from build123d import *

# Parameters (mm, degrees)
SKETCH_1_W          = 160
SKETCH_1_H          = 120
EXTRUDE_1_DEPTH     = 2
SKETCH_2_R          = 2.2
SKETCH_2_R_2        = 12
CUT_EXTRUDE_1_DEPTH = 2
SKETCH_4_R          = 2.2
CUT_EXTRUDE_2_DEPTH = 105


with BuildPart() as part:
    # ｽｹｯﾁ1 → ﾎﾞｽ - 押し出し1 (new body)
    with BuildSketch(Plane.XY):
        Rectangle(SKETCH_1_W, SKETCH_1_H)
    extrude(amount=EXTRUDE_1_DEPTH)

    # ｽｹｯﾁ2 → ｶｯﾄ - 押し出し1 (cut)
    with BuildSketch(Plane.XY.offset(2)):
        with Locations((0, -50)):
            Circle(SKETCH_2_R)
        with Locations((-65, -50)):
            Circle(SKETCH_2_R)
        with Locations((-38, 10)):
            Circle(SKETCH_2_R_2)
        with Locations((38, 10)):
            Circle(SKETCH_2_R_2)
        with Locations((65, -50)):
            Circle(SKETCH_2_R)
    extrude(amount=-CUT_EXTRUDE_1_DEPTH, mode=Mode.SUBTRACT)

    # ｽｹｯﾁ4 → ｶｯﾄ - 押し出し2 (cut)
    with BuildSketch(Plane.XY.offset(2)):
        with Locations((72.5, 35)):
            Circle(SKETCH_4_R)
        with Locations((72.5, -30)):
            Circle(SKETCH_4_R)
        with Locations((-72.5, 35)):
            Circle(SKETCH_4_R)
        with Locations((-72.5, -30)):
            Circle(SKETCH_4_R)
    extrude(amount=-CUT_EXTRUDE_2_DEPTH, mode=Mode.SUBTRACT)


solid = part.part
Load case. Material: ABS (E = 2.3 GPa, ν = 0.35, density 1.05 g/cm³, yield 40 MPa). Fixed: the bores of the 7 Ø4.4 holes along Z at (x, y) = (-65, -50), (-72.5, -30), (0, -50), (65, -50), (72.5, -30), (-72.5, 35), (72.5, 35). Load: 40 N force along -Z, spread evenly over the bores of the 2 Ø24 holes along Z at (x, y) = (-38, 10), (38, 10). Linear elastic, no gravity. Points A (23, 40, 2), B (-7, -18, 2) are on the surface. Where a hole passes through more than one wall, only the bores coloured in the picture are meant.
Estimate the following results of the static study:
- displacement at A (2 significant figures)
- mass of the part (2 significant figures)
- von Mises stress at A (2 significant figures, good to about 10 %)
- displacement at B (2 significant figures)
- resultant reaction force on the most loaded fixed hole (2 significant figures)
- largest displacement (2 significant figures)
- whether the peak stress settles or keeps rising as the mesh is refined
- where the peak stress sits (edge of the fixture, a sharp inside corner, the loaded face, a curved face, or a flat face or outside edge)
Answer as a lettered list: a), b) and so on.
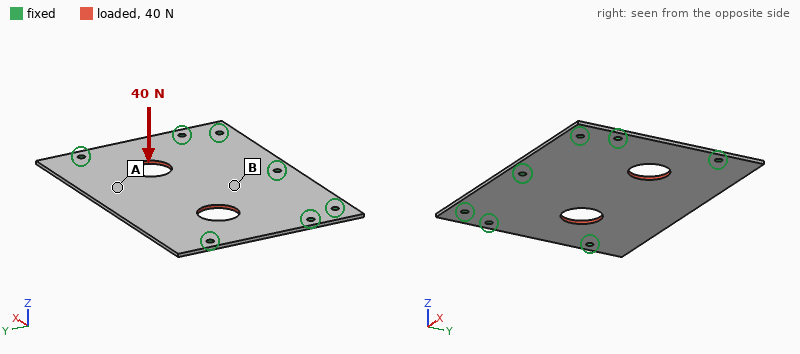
a) 1.7 mm
b) 38 g
c) 2.8 MPa
d) 1.0 mm
e) 12 N
f) 2.0 mm
g) keeps rising
h) edge of the fixture
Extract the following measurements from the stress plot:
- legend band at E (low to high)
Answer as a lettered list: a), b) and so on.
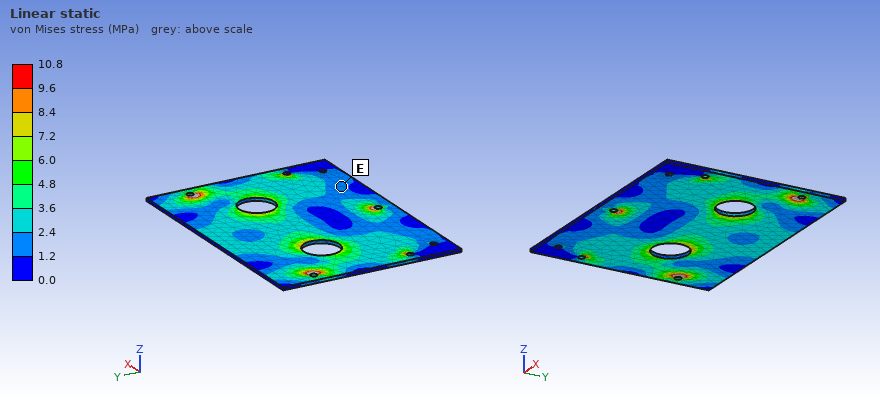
a) 1.2 to 2.4 MPa
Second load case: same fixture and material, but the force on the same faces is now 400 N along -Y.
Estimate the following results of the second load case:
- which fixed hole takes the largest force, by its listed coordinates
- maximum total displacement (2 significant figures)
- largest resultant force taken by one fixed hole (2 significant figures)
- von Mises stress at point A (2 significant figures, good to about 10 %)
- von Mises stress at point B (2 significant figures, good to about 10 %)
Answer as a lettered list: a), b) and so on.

a) (0, -50)
b) 51 µm
c) 110 N
d) 0.55 MPa
e) 1.0 MPa
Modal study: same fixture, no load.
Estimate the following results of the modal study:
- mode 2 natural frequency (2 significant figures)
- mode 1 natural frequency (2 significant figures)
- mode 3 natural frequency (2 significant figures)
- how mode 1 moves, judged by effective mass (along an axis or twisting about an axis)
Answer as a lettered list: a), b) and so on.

a) 300 Hz
b) 150 Hz
c) 380 Hz
d) along Z
